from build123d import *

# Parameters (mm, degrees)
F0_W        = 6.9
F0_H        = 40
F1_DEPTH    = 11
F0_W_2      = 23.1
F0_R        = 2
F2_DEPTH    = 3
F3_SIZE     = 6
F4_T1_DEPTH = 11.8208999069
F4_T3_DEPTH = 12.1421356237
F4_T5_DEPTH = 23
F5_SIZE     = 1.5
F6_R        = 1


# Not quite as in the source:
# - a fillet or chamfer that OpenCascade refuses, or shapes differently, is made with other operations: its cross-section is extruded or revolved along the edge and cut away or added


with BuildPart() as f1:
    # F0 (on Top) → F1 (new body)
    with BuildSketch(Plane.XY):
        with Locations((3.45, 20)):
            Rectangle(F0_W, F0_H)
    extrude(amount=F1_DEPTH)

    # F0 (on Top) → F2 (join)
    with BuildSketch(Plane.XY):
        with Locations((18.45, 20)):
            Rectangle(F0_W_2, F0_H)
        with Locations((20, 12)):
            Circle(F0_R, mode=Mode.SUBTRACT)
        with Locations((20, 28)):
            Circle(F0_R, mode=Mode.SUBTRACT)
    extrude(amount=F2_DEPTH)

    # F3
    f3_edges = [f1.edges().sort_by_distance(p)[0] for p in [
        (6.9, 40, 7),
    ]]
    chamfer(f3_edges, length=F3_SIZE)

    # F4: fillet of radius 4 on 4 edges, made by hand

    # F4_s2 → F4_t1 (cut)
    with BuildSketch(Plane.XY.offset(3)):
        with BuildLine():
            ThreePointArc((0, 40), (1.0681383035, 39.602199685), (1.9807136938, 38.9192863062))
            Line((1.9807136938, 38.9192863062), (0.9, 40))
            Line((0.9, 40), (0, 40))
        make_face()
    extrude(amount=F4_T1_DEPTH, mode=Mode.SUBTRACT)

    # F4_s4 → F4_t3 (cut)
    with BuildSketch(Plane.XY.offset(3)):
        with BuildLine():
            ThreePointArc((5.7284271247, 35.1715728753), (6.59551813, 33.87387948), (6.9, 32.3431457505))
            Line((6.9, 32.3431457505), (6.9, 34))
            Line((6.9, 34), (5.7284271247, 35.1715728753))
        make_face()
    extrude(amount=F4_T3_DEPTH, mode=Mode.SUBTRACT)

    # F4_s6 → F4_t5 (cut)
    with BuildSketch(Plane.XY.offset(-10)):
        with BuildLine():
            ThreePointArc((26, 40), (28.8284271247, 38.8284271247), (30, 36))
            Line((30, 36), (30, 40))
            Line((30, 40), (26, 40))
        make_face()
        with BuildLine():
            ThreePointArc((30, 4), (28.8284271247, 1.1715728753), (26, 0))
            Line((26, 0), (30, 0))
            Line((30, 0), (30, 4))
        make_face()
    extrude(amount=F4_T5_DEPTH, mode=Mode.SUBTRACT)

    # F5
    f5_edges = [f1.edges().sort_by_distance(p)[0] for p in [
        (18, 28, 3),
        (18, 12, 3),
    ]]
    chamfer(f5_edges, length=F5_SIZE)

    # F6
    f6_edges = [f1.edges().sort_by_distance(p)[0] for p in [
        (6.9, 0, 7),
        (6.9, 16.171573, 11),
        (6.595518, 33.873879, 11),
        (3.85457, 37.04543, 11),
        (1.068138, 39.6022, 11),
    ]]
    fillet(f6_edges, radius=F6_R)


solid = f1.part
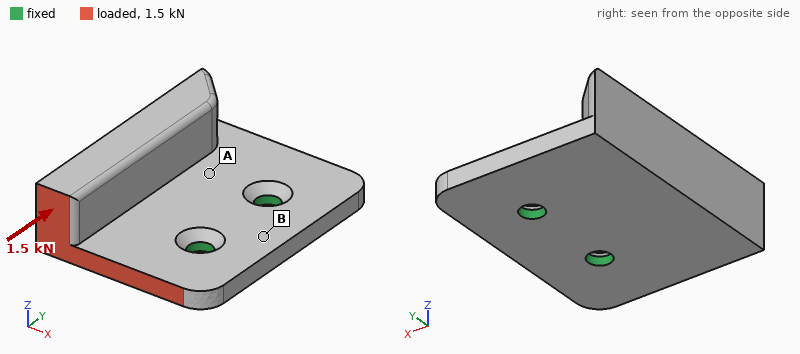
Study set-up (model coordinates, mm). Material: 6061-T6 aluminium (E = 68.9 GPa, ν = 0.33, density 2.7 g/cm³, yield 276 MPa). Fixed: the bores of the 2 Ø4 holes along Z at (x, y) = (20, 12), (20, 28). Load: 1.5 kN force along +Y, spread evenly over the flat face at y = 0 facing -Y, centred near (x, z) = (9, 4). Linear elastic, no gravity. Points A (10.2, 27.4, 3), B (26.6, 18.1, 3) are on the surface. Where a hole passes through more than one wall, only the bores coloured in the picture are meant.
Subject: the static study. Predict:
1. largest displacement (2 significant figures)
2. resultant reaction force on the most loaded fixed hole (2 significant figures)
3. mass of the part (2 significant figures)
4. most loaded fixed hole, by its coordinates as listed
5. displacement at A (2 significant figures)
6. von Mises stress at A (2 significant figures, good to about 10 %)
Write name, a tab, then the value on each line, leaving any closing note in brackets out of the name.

largest displacement	52 µm
resultant reaction force on the most loaded fixed hole	1.3 kN
mass of the part	15 g
most loaded fixed hole, by its coordinates as listed	(20, 12)
displacement at A	13 µm
von Mises stress at A	38 MPa
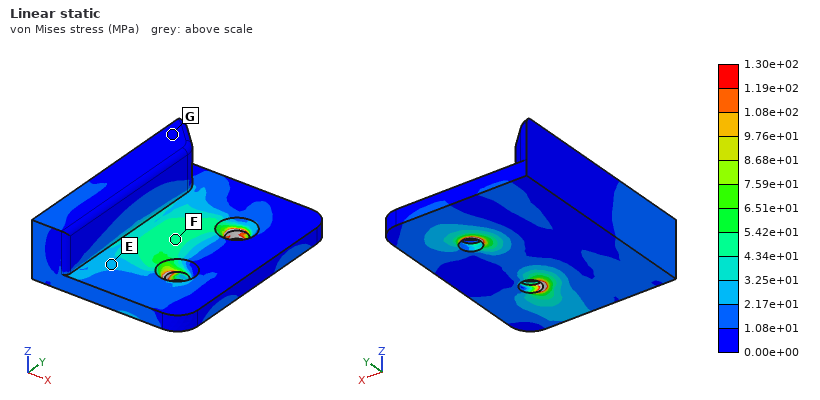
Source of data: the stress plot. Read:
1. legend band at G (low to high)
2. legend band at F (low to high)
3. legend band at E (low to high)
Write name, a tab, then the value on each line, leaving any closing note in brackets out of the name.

legend band at G	0.00e+00 to 1.08e+01 MPa
legend band at F	4.34e+01 to 5.42e+01 MPa
legend band at E	2.17e+01 to 3.25e+01 MPa
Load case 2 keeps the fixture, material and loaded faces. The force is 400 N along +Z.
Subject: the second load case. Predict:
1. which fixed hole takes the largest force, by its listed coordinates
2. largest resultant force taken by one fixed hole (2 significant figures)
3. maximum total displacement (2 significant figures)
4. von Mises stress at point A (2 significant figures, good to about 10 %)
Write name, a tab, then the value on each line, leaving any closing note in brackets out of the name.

which fixed hole takes the largest force, by its listed coordinates	(20, 12)
largest resultant force taken by one fixed hole	580 N
maximum total displacement	0.23 mm
von Mises stress at point A	51 MPa
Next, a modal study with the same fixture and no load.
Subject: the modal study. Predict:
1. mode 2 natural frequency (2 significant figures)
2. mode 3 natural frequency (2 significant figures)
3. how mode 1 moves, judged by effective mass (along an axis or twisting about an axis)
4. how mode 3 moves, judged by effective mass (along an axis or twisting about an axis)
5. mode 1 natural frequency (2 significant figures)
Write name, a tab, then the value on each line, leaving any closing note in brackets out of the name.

mode 2 natural frequency	5300 Hz
mode 3 natural frequency	13 kHz
how mode 1 moves, judged by effective mass	along Z
how mode 3 moves, judged by effective mass	along Y
mode 1 natural frequency	2600 Hz
